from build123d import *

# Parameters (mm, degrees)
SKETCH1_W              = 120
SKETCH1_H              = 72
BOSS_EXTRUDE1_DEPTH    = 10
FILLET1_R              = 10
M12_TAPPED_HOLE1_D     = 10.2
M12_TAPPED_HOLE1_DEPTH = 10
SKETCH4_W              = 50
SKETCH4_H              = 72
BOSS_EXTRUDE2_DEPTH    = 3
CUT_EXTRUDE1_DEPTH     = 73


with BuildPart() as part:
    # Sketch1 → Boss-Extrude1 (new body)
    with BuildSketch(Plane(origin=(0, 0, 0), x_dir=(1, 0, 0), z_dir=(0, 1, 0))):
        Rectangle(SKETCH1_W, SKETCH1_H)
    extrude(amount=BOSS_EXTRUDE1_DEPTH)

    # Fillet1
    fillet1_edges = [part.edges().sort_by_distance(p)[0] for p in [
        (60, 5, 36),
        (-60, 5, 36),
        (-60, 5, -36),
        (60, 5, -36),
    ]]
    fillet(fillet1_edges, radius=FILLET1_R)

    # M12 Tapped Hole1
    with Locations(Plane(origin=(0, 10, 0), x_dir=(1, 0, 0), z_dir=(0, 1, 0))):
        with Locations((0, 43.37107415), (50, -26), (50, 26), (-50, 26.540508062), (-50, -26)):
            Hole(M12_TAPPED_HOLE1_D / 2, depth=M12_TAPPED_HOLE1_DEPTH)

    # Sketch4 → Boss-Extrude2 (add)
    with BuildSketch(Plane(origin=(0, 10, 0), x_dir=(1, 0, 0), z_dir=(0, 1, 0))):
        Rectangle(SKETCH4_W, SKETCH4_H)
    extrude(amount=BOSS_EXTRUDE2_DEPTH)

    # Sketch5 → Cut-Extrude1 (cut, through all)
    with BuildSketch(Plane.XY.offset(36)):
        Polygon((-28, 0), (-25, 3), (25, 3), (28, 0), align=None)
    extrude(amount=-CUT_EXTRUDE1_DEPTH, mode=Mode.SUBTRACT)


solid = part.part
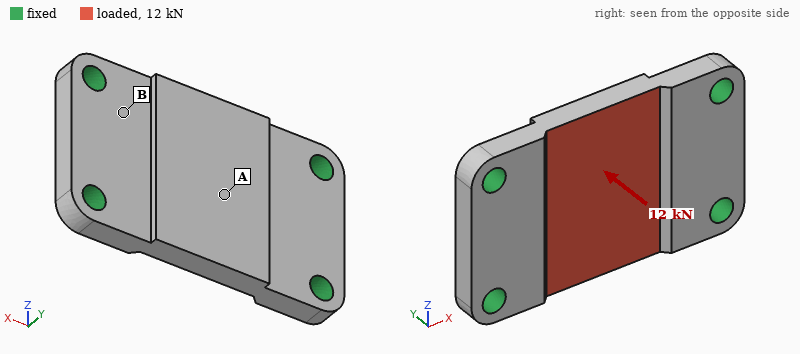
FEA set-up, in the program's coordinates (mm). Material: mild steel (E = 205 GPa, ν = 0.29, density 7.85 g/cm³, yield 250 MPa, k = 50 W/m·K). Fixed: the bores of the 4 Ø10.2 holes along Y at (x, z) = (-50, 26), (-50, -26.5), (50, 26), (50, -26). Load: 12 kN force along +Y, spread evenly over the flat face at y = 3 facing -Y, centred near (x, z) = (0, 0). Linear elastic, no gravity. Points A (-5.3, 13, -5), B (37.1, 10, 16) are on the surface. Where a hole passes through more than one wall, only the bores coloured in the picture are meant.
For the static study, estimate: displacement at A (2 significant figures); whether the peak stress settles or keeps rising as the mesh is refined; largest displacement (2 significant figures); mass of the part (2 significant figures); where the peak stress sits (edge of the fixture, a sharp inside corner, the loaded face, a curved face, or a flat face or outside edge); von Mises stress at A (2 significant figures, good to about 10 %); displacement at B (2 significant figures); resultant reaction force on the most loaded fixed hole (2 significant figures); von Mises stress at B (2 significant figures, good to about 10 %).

38 µm
keeps rising
39 µm
640 g
edge of the fixture
60 MPa
9.7 µm
4.9 kN
26 MPa
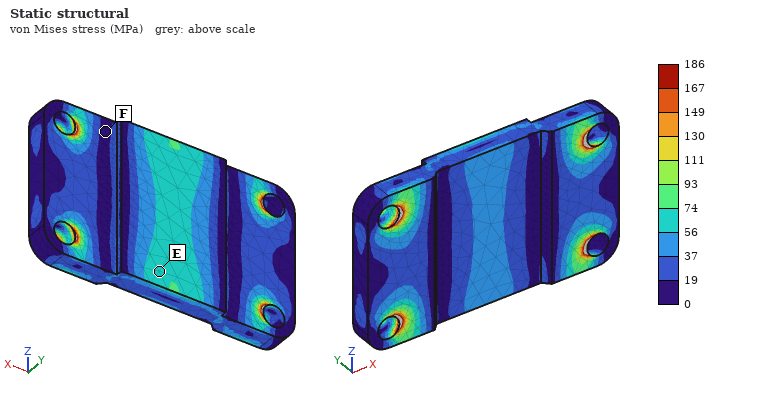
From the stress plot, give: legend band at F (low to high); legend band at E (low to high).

0 to 19 MPa
56 to 74 MPa
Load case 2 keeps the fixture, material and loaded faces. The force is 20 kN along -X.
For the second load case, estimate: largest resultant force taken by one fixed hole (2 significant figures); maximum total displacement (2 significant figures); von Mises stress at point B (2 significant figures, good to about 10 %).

5.1 kN
5.0 µm
21 MPa
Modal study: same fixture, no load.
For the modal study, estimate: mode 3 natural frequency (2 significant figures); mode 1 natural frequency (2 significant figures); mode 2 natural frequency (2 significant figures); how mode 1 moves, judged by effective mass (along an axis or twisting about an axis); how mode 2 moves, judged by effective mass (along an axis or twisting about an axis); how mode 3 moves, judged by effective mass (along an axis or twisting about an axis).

12 kHz
5300 Hz
7200 Hz
along Y
twisting about X
twisting about Z
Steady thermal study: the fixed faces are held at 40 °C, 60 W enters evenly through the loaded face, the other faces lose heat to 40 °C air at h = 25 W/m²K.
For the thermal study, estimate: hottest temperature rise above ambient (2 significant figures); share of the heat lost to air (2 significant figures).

33 K
10.0 %
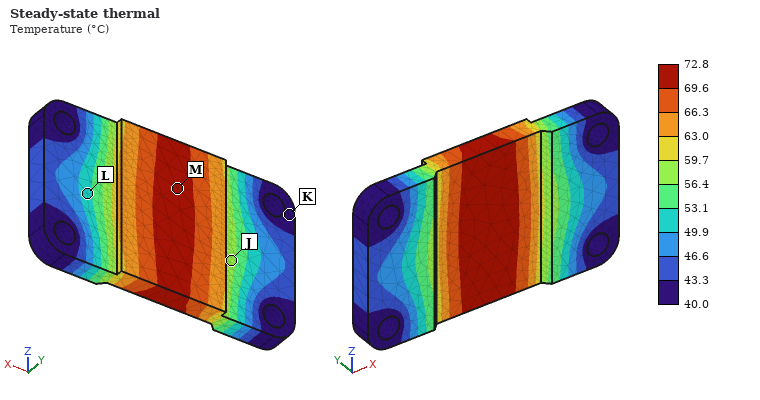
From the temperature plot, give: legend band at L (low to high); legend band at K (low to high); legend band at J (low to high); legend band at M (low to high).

49.9 to 53.1 °C
40.0 to 43.3 °C
56.4 to 59.7 °C
69.6 to 72.8 °C
